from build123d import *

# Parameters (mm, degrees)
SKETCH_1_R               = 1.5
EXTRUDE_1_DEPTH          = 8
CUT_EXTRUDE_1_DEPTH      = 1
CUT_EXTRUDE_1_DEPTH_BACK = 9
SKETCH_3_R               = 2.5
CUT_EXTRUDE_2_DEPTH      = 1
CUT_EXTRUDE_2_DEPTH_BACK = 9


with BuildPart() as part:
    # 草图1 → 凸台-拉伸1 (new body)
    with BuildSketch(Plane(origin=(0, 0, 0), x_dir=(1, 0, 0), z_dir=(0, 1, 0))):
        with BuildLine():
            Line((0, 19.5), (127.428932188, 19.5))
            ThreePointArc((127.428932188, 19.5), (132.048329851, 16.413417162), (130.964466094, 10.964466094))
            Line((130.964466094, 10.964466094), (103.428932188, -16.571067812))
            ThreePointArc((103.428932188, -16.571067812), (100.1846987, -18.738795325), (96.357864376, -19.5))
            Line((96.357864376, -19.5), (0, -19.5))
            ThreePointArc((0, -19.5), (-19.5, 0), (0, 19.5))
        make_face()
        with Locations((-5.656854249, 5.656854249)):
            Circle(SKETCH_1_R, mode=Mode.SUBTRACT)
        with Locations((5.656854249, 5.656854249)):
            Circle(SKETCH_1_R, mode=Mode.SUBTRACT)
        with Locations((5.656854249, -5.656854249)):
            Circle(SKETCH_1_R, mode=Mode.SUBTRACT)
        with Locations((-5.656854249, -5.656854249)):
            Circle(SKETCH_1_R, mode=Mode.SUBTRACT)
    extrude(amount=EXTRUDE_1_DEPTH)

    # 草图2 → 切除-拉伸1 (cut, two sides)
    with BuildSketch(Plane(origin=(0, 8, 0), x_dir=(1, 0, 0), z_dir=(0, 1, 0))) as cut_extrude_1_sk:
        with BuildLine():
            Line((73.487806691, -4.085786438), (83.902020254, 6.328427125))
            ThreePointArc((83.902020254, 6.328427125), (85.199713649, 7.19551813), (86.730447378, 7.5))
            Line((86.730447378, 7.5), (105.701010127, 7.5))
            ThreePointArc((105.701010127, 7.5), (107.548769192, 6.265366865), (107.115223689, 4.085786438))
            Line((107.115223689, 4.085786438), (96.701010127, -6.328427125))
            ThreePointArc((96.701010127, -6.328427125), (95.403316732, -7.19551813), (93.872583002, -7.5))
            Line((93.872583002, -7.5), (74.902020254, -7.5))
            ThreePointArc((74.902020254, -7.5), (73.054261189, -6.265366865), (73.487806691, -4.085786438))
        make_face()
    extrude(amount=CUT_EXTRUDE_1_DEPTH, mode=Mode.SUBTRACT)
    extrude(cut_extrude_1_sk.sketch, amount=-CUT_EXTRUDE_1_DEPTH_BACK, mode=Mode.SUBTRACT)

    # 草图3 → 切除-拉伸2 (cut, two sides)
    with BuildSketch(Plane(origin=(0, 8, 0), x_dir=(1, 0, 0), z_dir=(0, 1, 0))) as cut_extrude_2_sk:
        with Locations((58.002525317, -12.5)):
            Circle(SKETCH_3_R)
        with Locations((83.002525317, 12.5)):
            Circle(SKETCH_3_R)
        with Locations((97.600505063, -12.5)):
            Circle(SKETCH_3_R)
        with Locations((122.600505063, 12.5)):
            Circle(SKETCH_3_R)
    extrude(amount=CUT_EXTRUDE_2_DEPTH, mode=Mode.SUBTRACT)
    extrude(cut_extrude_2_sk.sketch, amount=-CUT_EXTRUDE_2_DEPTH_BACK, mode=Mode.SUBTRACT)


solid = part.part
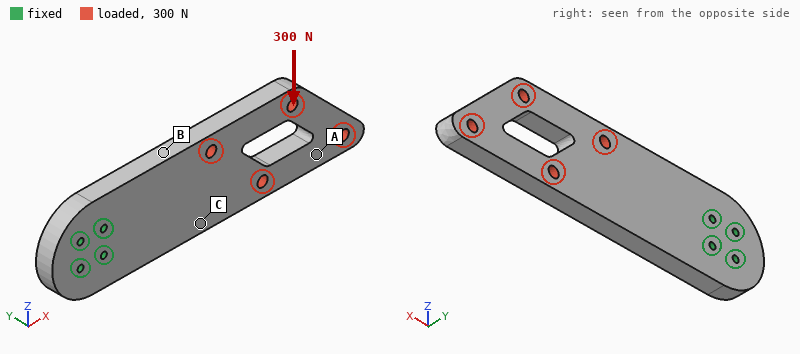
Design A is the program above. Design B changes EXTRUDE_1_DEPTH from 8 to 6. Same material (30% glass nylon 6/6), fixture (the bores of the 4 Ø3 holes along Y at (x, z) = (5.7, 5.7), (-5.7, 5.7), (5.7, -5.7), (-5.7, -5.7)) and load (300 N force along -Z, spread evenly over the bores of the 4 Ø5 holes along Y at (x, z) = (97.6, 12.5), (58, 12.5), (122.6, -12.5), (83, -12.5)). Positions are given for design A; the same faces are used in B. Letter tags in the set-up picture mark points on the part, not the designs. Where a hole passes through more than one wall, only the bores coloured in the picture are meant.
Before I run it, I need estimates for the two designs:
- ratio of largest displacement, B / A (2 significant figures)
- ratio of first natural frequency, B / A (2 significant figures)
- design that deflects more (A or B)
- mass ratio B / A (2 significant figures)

1.3
0.76
B
0.75
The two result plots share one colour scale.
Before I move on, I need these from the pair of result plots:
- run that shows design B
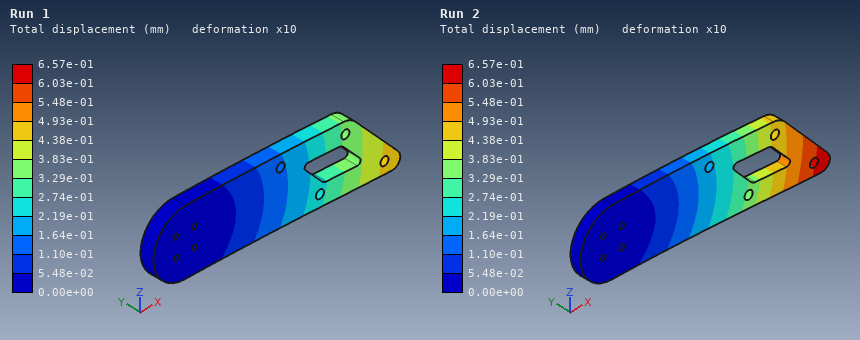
Run 2
